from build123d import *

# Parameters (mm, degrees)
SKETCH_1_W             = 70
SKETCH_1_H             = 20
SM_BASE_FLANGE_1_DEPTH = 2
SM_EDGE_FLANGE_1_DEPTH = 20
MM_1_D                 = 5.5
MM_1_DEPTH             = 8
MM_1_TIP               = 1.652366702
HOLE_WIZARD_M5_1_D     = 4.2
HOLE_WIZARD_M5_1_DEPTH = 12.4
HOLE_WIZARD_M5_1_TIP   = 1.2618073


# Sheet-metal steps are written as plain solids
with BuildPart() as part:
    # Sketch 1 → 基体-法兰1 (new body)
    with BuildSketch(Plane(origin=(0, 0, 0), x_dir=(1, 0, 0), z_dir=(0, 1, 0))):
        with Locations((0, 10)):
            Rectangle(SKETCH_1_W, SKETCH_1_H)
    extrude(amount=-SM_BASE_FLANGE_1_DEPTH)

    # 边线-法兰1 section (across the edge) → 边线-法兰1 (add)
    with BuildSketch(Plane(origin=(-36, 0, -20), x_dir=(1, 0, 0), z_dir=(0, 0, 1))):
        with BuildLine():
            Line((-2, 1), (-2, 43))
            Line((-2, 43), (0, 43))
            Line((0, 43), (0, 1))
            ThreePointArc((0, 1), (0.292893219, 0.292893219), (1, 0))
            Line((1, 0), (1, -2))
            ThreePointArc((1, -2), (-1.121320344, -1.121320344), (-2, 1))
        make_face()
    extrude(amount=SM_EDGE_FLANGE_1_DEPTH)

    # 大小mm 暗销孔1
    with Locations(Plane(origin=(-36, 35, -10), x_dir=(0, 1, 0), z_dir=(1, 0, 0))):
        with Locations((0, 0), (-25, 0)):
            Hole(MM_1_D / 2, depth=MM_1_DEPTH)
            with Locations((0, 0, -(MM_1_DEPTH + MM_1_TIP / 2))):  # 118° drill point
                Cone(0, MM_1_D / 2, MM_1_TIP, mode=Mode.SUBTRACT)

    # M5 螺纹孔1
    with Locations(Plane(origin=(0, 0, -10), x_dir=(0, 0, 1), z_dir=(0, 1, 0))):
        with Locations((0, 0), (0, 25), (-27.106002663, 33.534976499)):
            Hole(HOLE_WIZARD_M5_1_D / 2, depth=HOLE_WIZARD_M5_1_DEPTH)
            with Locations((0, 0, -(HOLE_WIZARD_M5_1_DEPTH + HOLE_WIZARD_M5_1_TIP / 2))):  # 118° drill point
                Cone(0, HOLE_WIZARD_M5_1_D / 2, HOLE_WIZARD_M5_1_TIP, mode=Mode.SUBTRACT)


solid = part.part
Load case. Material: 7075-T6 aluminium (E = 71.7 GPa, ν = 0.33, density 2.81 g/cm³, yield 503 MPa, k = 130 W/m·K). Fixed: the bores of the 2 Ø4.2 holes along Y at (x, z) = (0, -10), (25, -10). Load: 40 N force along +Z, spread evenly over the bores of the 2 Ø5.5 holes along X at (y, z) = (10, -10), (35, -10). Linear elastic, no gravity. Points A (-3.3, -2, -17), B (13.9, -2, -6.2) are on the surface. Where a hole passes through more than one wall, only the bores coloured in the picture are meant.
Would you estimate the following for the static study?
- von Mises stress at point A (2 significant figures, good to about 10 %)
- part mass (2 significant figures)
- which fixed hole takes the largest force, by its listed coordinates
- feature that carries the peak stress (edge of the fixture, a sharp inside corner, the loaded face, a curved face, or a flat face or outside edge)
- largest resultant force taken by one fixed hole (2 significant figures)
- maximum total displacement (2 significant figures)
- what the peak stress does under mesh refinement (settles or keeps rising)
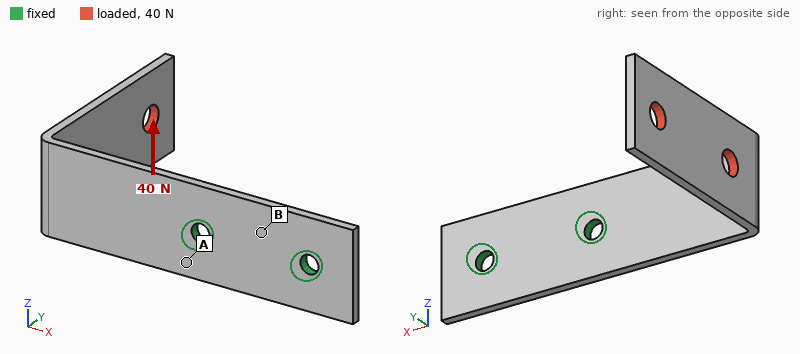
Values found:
46 MPa
13 g
(0, -10)
edge of the fixture
82 N
1.0 mm
keeps rising
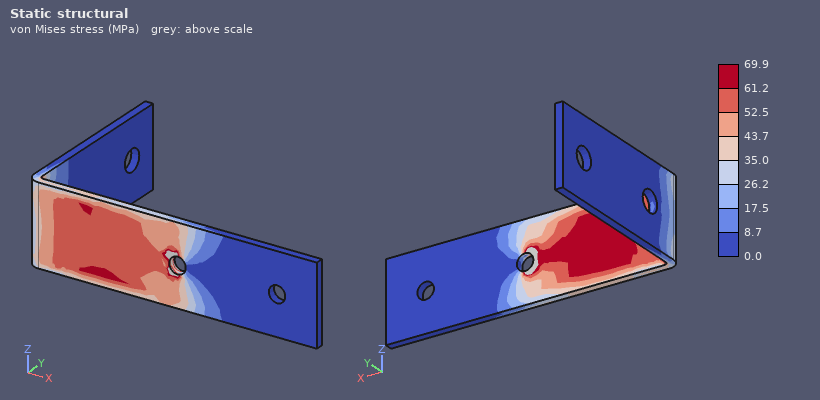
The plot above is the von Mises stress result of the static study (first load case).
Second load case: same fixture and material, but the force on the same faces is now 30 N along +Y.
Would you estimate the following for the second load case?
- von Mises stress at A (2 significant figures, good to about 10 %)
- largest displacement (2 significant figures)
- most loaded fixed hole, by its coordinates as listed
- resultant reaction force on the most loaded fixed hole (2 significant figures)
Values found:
57 MPa
1.0 mm
(0, -10)
34 N
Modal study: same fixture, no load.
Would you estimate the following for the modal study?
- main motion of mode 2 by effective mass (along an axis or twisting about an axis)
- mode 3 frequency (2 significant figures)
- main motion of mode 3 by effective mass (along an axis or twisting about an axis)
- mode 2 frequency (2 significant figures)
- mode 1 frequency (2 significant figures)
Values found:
along Z
960 Hz
along Y
570 Hz
350 Hz
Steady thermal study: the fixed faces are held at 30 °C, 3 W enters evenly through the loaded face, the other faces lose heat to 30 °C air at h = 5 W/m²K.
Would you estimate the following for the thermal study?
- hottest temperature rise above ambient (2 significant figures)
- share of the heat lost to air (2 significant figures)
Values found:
33 K
11 %
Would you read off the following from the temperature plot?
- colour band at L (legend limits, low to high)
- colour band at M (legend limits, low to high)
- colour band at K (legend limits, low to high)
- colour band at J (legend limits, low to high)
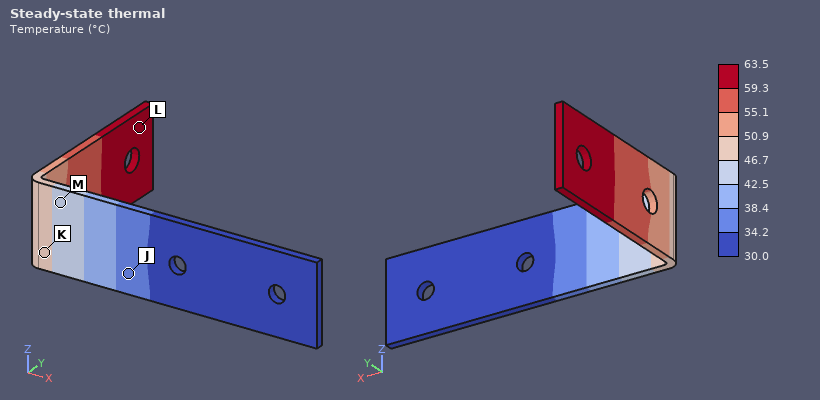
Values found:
59.3 to 63.5 °C
42.5 to 46.7 °C
46.7 to 50.9 °C
34.2 to 38.4 °C
